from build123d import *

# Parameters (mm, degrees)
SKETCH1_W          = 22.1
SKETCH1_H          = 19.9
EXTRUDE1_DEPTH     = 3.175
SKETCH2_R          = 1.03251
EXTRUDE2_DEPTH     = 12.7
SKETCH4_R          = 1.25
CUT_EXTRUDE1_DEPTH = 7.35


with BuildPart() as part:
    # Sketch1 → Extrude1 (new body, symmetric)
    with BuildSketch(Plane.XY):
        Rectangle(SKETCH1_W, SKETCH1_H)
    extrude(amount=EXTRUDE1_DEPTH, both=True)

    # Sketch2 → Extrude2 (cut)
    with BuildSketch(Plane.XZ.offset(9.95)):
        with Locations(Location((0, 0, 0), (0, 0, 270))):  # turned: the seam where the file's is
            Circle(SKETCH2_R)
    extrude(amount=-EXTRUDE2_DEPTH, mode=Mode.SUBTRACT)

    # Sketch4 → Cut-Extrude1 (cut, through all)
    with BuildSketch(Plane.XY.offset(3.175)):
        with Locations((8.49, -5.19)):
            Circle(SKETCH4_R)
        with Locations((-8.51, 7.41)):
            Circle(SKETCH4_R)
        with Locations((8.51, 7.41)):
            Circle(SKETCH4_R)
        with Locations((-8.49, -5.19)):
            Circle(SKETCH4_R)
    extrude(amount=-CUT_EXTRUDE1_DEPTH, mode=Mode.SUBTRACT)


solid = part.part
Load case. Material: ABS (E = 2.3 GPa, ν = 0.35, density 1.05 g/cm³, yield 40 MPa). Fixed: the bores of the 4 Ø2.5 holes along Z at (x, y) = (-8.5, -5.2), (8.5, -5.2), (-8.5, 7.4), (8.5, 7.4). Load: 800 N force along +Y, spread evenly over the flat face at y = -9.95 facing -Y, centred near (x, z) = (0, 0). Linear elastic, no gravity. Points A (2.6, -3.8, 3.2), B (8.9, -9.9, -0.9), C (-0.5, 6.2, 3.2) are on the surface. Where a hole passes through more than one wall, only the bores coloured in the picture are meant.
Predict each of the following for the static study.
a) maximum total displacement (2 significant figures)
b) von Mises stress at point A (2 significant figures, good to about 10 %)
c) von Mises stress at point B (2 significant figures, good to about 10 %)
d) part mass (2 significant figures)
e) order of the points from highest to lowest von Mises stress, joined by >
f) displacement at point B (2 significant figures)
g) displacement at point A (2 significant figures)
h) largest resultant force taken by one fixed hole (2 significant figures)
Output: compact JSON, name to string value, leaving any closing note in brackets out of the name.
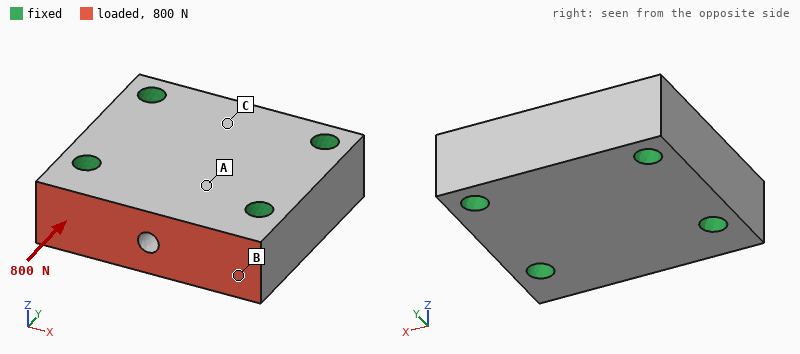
{"maximum total displacement": "31 µm", "von Mises stress at point A": "4.1 MPa", "von Mises stress at point B": "7.4 MPa", "part mass": "2.8 g", "order of the points from highest to lowest von Mises stress, joined by >": "B > A > C", "displacement at point B": "11 µm", "displacement at point A": "17 µm", "largest resultant force taken by one fixed hole": "320 N"}
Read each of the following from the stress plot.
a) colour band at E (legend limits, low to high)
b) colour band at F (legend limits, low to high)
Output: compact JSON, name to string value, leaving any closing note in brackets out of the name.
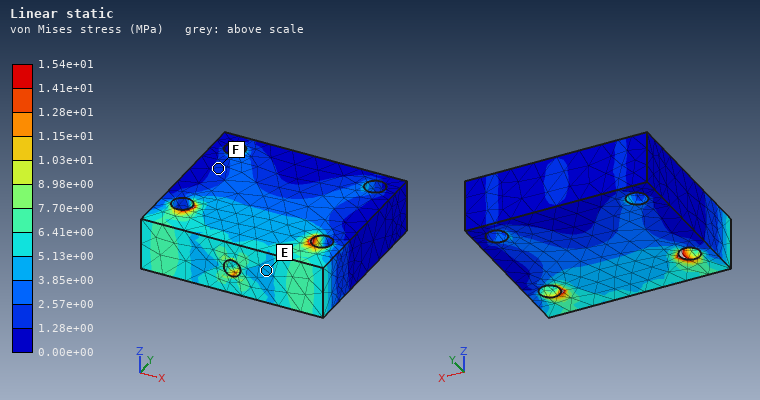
{"colour band at E": "3.85e+00 to 5.13e+00 MPa", "colour band at F": "1.28e+00 to 2.57e+00 MPa"}
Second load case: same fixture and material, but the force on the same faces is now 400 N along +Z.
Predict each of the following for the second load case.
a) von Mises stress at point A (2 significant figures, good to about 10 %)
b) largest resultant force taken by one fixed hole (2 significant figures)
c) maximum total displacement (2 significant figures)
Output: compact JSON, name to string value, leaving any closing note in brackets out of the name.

{"von Mises stress at point A": "5.9 MPa", "largest resultant force taken by one fixed hole": "220 N", "maximum total displacement": "77 µm"}
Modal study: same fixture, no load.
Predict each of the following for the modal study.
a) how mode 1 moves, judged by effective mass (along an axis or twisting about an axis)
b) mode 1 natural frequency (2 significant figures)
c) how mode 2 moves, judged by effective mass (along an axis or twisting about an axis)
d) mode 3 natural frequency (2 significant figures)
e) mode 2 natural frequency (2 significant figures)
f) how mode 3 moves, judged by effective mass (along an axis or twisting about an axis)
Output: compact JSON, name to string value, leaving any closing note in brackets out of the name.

{"how mode 1 moves, judged by effective mass": "along Z", "mode 1 natural frequency": "19 kHz", "how mode 2 moves, judged by effective mass": "twisting about X", "mode 3 natural frequency": "24 kHz", "mode 2 natural frequency": "22 kHz", "how mode 3 moves, judged by effective mass": "along Y"}
